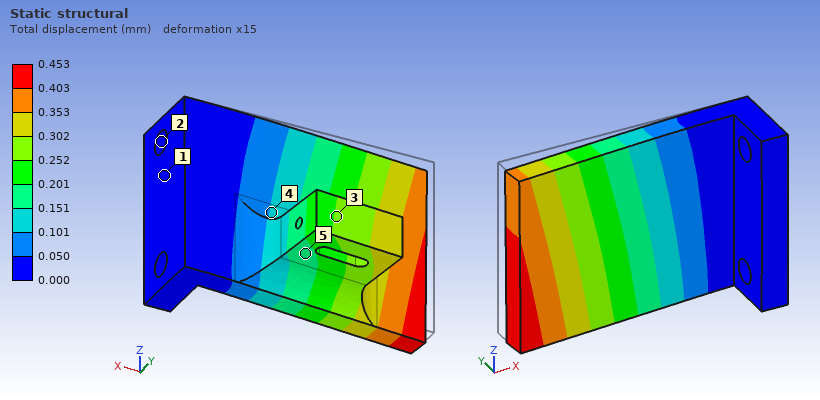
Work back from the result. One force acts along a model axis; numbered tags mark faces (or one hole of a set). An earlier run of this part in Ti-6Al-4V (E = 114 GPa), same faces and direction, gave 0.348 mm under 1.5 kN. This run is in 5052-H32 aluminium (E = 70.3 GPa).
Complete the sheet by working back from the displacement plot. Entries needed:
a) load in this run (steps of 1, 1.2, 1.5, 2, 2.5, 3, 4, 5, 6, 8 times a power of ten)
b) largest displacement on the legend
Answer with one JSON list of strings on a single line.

["1.2 kN", "0.453 mm"]
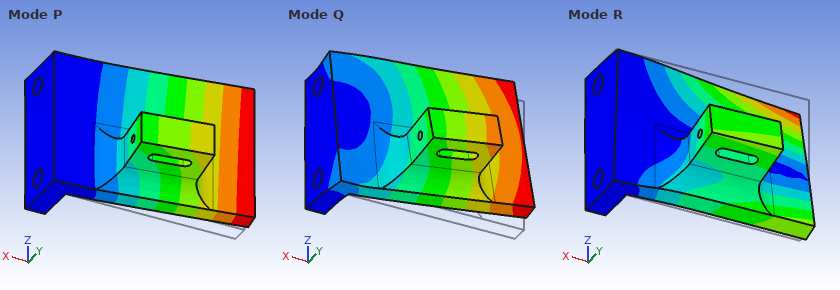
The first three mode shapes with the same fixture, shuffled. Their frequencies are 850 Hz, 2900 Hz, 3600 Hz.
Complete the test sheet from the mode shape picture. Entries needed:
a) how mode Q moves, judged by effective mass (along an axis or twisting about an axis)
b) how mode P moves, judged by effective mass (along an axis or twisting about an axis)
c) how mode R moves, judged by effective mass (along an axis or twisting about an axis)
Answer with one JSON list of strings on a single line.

["along Z", "along Y", "twisting about X"]
